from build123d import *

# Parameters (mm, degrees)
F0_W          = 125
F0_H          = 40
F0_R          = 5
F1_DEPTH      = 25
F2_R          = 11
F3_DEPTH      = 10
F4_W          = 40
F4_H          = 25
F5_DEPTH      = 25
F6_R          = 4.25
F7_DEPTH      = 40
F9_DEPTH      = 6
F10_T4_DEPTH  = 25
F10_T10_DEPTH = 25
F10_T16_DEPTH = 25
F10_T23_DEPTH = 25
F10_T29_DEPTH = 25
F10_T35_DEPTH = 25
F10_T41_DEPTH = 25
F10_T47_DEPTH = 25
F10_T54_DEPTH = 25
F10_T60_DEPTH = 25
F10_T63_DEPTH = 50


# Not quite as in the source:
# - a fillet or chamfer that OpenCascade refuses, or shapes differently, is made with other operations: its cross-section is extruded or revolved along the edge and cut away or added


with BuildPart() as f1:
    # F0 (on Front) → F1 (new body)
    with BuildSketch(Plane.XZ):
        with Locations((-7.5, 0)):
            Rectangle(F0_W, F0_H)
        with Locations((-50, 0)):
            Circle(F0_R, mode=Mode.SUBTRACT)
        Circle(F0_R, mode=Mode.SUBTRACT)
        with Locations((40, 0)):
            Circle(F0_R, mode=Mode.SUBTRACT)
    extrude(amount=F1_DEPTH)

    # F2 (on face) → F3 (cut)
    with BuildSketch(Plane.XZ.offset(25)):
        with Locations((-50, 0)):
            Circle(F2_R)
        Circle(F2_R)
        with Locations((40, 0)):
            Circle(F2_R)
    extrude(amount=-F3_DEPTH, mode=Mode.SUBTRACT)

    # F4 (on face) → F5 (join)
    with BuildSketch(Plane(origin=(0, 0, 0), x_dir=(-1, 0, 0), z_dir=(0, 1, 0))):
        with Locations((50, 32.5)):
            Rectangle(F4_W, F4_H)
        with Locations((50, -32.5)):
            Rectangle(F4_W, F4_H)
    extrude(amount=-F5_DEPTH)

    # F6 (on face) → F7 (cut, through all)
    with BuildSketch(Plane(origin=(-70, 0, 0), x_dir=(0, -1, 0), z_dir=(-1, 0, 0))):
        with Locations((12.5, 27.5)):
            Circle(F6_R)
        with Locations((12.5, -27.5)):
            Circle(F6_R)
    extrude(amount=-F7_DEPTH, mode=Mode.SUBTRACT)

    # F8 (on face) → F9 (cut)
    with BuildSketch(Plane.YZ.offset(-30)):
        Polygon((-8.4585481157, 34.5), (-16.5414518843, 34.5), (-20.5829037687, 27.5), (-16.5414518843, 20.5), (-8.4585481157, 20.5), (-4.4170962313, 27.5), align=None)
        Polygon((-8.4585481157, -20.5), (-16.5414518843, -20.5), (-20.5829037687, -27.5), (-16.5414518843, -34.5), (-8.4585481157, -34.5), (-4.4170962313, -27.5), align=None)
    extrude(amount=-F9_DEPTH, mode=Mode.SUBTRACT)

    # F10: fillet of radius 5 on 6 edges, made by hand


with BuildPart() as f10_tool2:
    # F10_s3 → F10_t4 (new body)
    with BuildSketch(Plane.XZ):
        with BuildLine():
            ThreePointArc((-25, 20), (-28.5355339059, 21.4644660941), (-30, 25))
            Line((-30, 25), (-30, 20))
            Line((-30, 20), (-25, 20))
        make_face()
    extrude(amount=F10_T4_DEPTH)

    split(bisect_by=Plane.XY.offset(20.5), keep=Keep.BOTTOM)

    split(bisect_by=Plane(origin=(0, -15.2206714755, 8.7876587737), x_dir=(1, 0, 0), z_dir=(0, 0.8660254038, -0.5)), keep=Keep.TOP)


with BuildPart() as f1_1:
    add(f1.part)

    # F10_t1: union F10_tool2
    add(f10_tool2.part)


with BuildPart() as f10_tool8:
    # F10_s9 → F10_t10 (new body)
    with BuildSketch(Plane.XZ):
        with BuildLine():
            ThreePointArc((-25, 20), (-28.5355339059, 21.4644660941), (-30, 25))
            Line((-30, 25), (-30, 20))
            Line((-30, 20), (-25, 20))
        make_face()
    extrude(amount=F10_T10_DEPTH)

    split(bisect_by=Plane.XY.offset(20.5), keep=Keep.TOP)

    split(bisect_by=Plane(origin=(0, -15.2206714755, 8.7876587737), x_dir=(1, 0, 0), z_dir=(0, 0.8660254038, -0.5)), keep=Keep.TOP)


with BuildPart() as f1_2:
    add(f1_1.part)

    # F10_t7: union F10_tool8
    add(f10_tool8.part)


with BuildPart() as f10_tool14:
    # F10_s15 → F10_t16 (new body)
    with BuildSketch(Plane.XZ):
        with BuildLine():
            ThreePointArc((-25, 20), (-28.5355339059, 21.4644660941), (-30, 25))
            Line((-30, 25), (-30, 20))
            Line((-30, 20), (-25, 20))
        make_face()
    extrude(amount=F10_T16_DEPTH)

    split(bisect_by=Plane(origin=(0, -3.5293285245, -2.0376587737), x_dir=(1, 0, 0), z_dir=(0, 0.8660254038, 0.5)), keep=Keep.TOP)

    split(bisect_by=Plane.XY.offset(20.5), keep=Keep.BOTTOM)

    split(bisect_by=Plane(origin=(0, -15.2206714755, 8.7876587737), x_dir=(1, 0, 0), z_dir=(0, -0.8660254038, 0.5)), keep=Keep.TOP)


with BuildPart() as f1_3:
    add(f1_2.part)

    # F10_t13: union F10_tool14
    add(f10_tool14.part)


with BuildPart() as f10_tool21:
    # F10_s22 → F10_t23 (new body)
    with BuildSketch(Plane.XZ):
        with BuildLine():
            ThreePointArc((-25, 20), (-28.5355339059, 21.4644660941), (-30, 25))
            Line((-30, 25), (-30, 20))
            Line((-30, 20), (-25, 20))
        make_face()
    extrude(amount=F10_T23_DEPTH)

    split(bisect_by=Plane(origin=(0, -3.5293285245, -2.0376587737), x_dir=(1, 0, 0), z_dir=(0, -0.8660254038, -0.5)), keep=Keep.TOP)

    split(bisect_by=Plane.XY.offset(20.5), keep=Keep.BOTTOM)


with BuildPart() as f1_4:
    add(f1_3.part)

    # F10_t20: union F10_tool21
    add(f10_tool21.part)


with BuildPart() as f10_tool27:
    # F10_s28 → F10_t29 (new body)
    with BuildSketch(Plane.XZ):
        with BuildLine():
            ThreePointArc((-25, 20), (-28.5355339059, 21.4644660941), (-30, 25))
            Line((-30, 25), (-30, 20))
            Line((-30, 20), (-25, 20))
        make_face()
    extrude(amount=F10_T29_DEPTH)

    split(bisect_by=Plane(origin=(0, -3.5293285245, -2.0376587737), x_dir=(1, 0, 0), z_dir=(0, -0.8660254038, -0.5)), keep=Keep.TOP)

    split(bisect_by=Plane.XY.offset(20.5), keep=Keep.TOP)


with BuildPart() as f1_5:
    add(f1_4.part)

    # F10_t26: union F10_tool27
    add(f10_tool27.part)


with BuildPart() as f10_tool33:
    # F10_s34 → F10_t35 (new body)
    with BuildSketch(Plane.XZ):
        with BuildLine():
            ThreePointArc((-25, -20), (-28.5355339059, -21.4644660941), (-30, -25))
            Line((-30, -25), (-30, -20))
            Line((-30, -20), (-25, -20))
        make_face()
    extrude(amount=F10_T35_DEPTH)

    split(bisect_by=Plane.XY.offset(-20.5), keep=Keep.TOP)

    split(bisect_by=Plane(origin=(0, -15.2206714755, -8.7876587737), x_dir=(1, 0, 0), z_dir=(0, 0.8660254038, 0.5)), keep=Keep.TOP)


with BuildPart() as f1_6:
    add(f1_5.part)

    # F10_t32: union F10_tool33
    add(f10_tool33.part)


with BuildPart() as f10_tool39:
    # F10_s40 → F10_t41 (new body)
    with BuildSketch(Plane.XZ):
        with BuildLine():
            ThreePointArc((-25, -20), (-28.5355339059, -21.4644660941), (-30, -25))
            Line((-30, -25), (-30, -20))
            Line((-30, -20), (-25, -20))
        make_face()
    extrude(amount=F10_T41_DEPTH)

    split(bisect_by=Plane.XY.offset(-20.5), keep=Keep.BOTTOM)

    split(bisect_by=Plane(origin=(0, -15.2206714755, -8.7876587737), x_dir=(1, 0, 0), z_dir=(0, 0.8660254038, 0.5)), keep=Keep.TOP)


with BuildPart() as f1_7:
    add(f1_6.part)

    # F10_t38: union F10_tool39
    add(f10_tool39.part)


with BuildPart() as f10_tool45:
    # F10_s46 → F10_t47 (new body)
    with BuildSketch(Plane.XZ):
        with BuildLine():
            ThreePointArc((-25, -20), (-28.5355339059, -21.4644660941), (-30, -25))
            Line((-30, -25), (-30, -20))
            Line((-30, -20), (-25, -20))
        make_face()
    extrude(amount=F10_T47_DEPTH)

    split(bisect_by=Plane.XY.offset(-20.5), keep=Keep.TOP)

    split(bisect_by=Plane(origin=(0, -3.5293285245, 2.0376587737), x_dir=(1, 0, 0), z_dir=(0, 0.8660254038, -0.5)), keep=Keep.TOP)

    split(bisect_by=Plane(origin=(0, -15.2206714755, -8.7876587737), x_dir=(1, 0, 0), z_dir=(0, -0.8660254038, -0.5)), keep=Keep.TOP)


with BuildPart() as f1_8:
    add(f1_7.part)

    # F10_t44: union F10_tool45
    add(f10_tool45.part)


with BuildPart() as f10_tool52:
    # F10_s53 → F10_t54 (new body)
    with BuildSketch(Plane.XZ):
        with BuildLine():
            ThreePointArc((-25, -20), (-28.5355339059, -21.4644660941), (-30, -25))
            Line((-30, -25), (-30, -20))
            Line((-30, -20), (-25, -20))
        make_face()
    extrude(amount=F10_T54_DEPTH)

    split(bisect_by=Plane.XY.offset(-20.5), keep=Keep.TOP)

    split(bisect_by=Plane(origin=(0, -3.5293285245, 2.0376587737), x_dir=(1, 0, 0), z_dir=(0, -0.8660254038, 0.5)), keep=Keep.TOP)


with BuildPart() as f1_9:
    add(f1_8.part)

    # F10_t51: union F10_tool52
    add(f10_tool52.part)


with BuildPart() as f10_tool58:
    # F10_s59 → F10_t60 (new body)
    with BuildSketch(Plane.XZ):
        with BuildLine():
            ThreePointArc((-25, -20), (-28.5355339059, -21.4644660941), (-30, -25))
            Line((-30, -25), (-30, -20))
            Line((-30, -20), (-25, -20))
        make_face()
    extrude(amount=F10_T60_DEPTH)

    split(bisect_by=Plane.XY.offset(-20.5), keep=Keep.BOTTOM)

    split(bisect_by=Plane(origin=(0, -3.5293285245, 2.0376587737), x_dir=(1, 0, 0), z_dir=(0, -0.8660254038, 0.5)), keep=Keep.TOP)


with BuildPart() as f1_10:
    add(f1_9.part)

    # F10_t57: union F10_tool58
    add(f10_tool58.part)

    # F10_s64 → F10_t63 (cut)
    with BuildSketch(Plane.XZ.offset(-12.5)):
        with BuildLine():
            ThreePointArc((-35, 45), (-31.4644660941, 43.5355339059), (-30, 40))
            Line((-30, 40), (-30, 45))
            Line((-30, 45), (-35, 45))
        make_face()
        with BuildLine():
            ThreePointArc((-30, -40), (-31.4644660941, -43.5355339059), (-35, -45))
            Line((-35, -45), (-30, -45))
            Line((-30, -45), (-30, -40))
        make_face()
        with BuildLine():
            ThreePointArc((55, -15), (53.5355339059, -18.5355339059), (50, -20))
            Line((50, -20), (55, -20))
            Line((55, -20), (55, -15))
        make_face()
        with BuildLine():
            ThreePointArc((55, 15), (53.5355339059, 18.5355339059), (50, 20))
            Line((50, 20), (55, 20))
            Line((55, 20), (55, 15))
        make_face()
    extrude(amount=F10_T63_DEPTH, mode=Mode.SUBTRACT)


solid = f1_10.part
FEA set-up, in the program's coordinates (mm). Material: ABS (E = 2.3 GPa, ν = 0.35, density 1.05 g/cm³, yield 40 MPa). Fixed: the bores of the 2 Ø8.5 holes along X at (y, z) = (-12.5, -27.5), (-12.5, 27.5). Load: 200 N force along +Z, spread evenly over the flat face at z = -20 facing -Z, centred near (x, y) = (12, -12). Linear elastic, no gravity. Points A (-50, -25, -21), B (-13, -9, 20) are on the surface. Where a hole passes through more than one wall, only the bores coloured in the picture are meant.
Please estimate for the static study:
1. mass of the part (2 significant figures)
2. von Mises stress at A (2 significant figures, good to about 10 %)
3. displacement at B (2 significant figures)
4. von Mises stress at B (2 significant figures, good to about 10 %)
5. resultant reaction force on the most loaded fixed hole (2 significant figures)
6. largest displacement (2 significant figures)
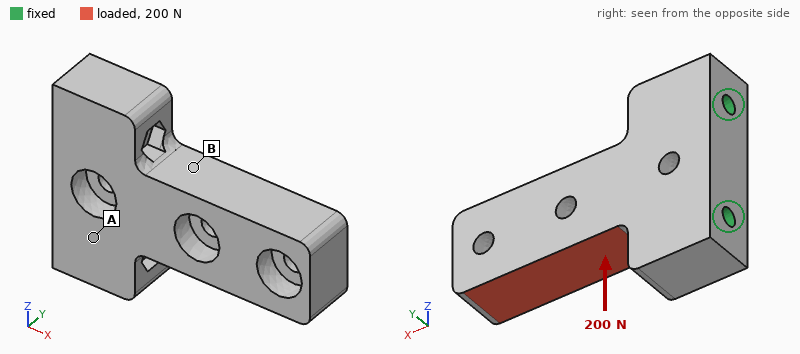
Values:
160 g
0.32 MPa
0.024 mm
0.99 MPa
250 N
0.11 mm
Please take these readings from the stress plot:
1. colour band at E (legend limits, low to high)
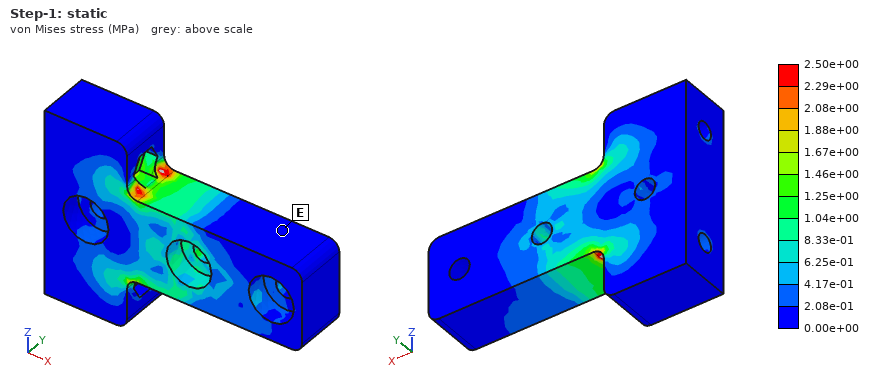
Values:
0.00e+00 to 2.08e-01 MPa
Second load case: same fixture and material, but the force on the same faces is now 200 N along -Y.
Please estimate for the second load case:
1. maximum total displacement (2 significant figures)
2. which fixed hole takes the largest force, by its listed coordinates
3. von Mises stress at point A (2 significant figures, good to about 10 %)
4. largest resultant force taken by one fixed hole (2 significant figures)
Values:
0.42 mm
(-12.5, -27.5)
1.5 MPa
180 N
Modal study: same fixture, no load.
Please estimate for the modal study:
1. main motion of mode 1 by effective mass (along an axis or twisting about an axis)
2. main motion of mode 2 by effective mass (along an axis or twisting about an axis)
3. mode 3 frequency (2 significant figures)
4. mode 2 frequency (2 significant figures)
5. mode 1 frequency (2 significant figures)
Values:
along Y
along Z
1800 Hz
960 Hz
510 Hz
